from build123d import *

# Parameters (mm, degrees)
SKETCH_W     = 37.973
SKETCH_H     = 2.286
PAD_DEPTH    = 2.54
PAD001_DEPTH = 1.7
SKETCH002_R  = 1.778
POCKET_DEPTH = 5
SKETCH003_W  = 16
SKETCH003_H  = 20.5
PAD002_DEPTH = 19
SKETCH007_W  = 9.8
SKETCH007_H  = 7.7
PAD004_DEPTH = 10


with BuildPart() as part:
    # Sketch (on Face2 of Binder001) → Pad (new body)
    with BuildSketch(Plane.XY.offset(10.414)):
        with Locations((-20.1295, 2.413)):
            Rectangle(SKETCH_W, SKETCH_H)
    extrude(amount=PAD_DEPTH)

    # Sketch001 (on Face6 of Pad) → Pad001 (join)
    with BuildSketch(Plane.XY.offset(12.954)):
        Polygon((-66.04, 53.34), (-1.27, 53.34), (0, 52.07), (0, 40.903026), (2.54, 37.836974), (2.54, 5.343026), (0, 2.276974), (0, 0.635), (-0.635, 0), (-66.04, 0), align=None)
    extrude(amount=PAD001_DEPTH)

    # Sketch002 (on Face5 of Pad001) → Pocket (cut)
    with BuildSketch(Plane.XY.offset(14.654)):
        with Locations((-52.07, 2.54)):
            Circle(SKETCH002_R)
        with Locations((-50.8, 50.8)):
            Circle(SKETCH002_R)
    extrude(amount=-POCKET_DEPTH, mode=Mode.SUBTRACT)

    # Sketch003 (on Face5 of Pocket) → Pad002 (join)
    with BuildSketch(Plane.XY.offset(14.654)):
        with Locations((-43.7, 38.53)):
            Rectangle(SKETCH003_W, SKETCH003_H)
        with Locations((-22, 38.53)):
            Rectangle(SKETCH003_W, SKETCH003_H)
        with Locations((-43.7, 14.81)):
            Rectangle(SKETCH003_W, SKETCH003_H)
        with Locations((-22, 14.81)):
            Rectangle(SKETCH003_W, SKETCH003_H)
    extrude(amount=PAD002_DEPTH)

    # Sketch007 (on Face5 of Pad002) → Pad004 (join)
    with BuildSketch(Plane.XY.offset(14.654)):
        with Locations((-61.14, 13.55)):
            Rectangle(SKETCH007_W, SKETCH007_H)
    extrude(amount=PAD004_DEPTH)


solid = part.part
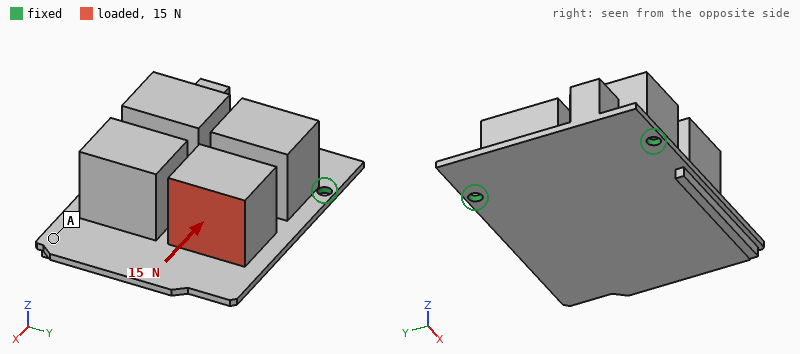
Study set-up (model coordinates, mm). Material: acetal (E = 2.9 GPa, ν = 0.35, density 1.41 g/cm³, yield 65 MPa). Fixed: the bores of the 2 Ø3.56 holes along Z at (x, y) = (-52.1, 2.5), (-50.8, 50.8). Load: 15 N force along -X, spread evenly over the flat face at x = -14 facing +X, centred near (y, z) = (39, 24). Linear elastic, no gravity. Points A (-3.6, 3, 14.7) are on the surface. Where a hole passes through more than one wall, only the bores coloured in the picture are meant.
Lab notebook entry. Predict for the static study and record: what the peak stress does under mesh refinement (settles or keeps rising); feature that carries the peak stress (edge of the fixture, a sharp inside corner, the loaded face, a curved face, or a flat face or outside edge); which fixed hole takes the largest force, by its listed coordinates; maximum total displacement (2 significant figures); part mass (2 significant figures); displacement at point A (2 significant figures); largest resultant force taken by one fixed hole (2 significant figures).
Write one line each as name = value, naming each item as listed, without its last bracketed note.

what the peak stress does under mesh refinement = keeps rising
feature that carries the peak stress = edge of the fixture
which fixed hole takes the largest force, by its listed coordinates = (-50.8, 50.8)
maximum total displacement = 0.85 mm
part mass = 45 g
displacement at point A = 0.70 mm
largest resultant force taken by one fixed hole = 11 N
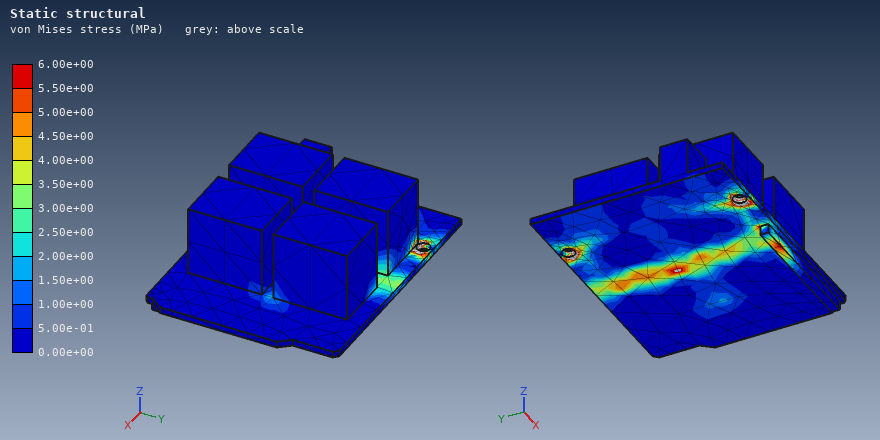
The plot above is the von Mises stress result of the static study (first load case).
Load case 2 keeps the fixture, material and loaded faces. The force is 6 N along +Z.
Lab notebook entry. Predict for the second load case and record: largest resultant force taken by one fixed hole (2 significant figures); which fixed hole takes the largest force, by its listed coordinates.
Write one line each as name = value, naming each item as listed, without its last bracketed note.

largest resultant force taken by one fixed hole = 4.8 N
which fixed hole takes the largest force, by its listed coordinates = (-50.8, 50.8)
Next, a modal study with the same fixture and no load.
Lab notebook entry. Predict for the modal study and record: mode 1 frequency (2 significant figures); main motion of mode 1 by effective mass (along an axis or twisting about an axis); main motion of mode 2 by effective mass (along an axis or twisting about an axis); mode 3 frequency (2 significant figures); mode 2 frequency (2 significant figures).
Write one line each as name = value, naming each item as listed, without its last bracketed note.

mode 1 frequency = 120 Hz
main motion of mode 1 by effective mass = along Z
main motion of mode 2 by effective mass = along Z
mode 3 frequency = 550 Hz
mode 2 frequency = 420 Hz
